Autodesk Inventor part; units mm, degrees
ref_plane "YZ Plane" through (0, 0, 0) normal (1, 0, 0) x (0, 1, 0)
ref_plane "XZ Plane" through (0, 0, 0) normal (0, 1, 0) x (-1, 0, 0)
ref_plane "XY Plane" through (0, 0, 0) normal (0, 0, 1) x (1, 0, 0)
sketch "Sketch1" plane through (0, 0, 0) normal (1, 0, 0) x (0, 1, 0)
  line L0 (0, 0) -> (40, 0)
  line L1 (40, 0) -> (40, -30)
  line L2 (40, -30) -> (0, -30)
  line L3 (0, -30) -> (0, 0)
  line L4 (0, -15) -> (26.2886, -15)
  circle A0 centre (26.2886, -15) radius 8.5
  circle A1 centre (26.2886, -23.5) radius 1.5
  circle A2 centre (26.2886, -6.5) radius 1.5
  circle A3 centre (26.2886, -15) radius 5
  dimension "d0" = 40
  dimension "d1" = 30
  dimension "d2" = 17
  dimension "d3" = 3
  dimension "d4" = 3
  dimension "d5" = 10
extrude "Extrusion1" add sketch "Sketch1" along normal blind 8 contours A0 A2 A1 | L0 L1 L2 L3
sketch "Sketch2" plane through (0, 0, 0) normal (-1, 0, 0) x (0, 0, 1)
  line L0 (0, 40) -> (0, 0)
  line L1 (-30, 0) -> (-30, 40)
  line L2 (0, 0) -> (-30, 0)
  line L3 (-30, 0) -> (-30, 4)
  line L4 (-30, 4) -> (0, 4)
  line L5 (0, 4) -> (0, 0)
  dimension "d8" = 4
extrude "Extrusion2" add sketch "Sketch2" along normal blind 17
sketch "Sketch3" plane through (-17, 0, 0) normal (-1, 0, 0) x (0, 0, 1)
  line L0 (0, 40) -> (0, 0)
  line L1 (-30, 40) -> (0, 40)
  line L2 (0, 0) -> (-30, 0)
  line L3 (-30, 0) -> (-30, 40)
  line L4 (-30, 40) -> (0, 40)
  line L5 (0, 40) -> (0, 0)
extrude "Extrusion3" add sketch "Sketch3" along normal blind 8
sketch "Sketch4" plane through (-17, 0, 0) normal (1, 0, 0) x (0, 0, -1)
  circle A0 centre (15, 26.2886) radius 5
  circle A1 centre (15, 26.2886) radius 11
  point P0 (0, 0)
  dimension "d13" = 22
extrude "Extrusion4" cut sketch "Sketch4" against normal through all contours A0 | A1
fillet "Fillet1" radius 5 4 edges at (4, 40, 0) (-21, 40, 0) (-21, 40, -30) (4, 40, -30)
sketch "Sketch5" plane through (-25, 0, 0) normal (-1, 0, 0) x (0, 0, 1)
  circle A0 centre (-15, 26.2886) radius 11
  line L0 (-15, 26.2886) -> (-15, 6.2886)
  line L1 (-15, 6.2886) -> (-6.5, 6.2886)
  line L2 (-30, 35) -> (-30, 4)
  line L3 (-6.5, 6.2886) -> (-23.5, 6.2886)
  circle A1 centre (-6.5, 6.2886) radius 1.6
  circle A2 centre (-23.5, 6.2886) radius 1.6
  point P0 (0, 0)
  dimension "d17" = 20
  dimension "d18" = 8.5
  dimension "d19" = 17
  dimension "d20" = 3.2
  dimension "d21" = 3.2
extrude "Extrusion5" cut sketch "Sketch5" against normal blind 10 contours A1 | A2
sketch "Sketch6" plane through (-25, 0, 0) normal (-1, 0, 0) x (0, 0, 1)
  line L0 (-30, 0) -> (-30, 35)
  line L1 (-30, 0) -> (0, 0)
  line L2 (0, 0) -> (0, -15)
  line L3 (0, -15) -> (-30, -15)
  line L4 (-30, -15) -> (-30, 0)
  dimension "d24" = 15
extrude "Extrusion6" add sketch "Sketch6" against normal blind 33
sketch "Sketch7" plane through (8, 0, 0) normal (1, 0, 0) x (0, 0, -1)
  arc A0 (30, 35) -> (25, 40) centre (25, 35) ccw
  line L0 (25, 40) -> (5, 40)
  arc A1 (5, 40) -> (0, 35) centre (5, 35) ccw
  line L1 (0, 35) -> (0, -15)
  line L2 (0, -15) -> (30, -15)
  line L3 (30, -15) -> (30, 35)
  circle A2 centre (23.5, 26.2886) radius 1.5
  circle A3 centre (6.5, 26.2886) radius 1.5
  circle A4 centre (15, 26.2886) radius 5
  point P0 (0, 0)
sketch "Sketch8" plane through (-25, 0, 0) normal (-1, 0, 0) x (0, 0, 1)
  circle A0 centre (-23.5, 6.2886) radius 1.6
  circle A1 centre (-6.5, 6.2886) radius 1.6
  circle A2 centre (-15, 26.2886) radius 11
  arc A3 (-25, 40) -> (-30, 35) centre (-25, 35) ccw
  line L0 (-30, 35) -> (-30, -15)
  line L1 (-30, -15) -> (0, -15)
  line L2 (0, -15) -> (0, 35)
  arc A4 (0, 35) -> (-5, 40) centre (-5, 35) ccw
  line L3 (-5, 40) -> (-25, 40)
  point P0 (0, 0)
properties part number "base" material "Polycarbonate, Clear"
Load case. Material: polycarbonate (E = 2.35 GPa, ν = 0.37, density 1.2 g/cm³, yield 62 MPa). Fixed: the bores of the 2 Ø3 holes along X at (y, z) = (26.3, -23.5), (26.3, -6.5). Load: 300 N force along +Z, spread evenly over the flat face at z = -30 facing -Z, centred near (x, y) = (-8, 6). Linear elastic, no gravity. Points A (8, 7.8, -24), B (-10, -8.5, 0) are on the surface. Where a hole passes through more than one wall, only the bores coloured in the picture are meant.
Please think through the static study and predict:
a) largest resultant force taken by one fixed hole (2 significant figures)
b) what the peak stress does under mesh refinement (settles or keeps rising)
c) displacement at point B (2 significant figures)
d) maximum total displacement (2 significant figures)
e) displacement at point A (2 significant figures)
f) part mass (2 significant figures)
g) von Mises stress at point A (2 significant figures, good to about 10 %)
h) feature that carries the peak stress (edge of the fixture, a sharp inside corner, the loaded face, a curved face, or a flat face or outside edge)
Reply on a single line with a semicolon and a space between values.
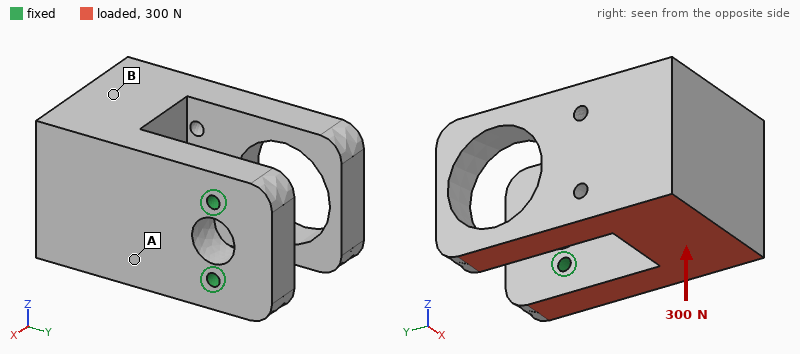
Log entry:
390 N; keeps rising; 0.43 mm; 0.68 mm; 0.12 mm; 38 g; 5.4 MPa; edge of the fixture
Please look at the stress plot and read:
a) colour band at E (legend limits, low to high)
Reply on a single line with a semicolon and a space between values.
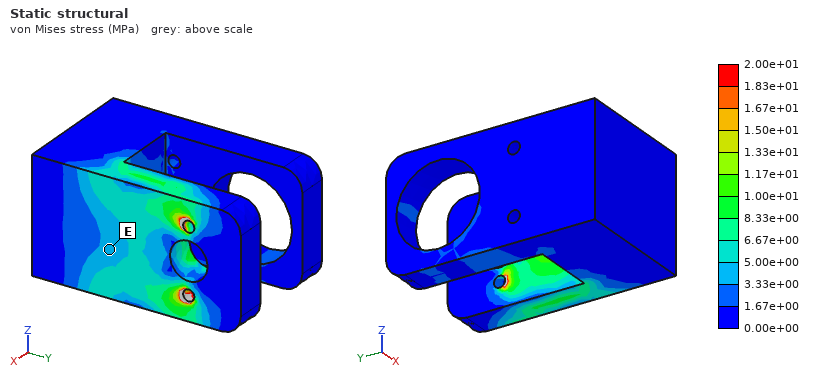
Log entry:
3.33e+00 to 5.00e+00 MPa
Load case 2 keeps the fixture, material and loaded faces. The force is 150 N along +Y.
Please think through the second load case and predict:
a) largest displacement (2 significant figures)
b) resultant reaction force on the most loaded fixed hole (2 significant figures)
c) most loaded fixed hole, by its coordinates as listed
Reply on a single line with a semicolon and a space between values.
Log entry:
0.78 mm; 200 N; (26.3, -23.5)
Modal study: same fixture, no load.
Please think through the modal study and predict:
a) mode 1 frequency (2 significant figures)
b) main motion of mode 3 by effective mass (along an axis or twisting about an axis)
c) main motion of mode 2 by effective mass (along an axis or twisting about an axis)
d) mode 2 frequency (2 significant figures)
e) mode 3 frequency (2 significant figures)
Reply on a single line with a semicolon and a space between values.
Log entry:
350 Hz; along X; along Z; 630 Hz; 980 Hz
